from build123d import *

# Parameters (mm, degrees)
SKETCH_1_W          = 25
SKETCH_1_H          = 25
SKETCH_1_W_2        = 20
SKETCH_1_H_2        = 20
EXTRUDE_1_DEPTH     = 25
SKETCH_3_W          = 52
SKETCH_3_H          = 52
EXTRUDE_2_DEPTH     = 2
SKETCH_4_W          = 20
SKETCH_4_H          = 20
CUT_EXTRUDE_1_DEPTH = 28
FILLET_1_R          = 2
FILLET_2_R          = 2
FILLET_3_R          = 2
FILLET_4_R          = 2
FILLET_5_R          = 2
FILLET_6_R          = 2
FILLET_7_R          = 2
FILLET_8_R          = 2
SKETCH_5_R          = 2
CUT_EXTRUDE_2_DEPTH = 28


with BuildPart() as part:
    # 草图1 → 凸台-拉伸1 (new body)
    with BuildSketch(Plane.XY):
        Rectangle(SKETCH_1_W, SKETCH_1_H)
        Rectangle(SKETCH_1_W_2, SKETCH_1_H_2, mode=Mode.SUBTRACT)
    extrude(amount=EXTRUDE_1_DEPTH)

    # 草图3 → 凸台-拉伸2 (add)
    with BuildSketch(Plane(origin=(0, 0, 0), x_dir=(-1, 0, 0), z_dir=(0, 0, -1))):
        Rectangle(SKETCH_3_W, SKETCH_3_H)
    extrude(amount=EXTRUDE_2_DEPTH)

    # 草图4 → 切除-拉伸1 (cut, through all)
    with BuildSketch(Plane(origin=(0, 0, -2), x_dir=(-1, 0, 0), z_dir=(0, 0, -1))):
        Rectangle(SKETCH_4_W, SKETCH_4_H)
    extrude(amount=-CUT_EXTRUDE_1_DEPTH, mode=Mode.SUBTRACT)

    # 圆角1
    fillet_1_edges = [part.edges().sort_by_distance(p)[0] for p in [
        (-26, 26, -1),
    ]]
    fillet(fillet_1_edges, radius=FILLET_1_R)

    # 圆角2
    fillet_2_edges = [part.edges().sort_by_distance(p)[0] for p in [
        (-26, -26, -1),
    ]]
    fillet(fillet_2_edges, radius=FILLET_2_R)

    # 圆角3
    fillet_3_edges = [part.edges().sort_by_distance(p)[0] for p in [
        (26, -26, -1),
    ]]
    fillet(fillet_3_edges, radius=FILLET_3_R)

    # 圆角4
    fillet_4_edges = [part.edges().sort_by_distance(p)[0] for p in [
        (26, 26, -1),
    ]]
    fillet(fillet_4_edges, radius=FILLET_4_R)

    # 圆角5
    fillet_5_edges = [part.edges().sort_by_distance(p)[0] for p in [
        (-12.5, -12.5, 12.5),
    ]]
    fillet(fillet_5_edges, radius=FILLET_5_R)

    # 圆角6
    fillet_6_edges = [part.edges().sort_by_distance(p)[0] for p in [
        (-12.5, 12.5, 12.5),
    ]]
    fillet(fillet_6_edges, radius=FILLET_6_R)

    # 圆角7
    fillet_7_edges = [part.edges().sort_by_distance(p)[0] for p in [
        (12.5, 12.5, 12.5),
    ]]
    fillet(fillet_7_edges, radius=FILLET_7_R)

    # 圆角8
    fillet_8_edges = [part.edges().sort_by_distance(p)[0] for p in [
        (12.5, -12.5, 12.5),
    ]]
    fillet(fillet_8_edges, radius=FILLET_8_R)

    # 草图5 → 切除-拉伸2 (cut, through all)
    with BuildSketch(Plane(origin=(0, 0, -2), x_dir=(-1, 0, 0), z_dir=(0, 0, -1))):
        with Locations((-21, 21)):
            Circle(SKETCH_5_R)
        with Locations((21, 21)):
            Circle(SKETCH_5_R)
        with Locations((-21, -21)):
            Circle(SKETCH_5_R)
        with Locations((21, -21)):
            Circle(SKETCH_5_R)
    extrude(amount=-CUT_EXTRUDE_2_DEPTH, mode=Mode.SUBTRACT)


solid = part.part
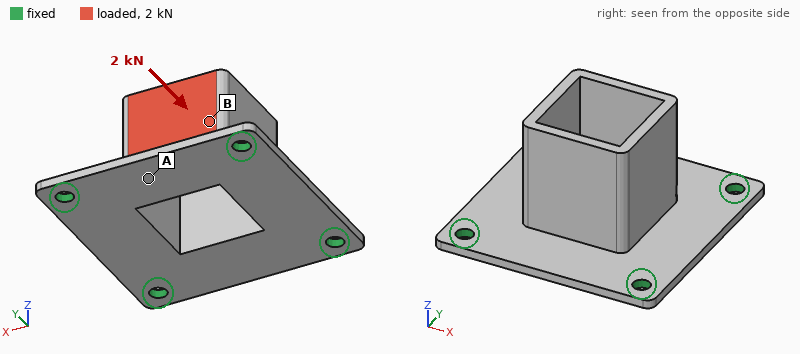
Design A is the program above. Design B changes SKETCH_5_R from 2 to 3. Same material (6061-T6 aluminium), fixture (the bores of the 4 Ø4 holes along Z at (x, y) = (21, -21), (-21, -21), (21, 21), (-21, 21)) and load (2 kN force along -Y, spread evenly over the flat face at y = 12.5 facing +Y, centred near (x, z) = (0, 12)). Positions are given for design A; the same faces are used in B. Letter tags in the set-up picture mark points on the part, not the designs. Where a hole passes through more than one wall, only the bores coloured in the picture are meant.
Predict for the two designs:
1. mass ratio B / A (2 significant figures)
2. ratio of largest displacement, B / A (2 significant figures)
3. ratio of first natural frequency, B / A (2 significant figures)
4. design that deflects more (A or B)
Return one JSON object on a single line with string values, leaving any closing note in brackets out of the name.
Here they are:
{"mass ratio B / A": "0.99", "ratio of largest displacement, B / A": "0.89", "ratio of first natural frequency, B / A": "1.1", "design that deflects more": "A"}
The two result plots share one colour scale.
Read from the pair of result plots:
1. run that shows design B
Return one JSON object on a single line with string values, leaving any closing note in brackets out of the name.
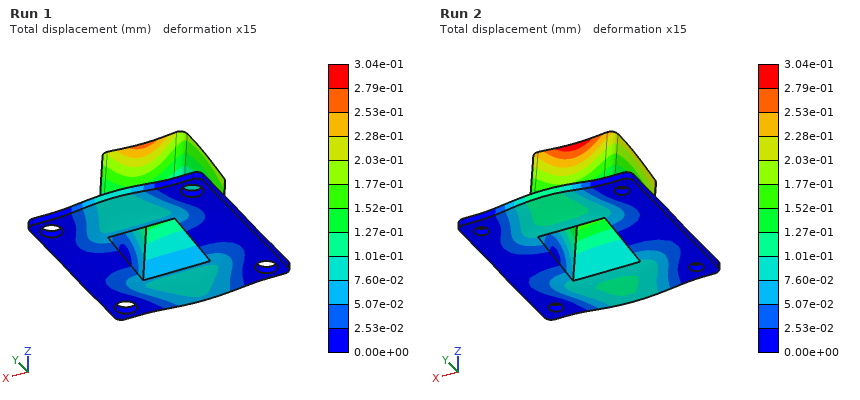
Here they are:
{"run that shows design B": "Run 1"}
